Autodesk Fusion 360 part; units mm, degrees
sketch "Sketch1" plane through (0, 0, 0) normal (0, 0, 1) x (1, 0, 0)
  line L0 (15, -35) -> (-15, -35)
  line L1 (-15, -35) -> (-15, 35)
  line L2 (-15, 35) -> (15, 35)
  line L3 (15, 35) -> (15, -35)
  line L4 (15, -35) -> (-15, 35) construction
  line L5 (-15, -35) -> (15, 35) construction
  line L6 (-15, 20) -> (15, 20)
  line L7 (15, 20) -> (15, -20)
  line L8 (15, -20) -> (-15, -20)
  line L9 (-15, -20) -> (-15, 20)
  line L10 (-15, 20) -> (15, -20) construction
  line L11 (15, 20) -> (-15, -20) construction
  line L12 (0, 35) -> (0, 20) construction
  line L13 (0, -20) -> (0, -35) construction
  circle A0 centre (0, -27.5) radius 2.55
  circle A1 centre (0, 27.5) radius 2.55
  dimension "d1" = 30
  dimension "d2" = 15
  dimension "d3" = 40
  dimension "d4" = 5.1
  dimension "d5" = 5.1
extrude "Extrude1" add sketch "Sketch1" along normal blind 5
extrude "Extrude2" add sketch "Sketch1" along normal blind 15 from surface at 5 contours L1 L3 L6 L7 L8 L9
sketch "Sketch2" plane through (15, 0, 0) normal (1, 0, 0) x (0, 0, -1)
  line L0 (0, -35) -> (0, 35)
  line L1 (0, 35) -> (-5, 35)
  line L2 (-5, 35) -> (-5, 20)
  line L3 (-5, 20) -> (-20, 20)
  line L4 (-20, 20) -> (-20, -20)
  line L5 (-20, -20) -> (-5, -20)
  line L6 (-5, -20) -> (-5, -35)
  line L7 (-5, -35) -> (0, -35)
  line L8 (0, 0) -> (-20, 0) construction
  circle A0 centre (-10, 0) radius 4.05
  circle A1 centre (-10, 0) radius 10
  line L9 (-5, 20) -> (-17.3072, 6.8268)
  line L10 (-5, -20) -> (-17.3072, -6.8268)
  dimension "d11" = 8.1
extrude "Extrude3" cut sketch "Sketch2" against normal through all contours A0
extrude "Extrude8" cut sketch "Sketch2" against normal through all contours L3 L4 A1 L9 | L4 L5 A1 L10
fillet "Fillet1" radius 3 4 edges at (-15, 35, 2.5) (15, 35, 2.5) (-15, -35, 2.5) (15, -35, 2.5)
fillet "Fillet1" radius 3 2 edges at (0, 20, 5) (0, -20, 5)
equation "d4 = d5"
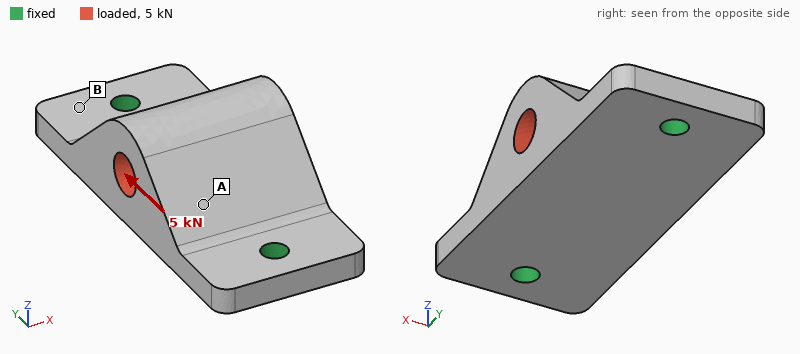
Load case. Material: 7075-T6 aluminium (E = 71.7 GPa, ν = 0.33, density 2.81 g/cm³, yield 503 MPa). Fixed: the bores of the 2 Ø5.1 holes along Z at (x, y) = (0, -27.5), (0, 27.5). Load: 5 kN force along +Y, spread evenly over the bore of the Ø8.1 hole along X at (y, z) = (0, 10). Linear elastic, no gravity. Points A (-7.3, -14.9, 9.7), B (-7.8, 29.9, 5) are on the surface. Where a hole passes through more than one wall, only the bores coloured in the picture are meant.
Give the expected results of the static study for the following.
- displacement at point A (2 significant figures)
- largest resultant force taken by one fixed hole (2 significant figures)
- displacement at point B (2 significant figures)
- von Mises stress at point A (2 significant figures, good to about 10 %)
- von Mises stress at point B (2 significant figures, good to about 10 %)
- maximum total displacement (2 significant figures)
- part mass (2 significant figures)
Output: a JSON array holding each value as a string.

["8.4 µm", "2.6 kN", "2.5 µm", "14 MPa", "6.2 MPa", "11 µm", "54 g"]
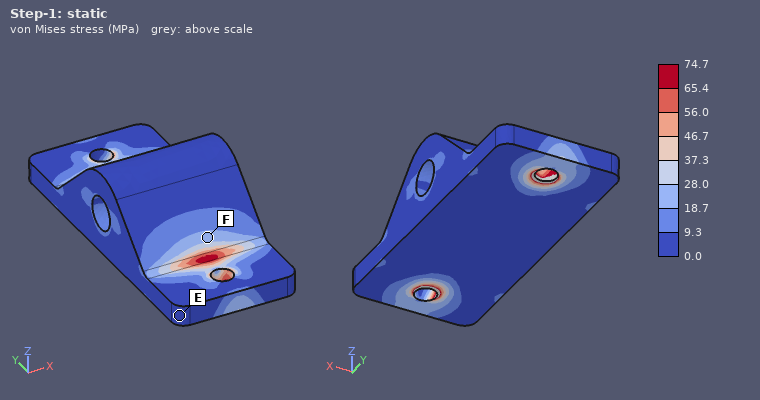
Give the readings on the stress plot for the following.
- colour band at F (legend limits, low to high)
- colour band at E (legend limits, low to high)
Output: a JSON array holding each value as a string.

["18.7 to 28.0 MPa", "0.0 to 9.3 MPa"]
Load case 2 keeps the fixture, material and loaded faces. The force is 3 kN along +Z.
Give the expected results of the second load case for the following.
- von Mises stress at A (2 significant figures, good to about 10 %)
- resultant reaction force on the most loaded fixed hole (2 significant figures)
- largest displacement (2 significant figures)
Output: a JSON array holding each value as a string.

["29 MPa", "1.9 kN", "26 µm"]
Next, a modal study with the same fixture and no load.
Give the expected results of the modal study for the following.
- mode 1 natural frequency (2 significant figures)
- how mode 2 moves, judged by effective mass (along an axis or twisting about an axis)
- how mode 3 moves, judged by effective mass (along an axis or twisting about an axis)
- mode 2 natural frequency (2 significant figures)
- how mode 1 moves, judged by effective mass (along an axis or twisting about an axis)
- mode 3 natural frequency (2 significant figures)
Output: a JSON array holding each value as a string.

["5400 Hz", "along Z", "along X", "9100 Hz", "along X", "15 kHz"]
